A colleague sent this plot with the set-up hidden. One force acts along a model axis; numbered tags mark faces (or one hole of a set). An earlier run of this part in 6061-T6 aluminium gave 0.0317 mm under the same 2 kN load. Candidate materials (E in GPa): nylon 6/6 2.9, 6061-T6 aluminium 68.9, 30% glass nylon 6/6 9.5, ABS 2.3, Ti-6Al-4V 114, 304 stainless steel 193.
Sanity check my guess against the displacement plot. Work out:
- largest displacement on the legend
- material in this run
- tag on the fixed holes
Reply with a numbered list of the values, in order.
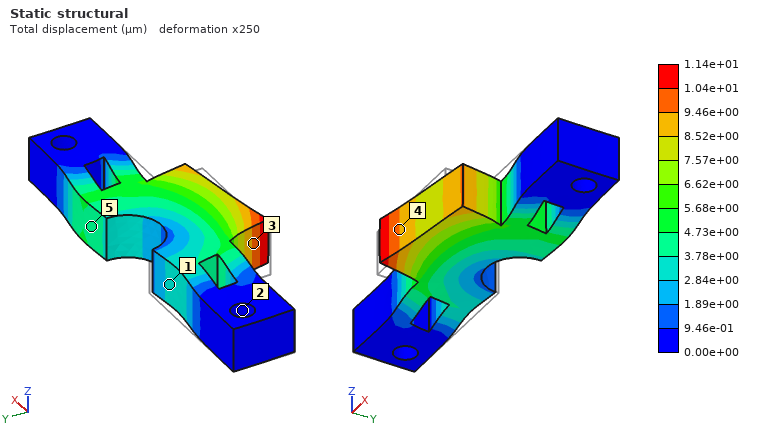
1. 1.14e+01 µm
2. 304 stainless steel
3. 2
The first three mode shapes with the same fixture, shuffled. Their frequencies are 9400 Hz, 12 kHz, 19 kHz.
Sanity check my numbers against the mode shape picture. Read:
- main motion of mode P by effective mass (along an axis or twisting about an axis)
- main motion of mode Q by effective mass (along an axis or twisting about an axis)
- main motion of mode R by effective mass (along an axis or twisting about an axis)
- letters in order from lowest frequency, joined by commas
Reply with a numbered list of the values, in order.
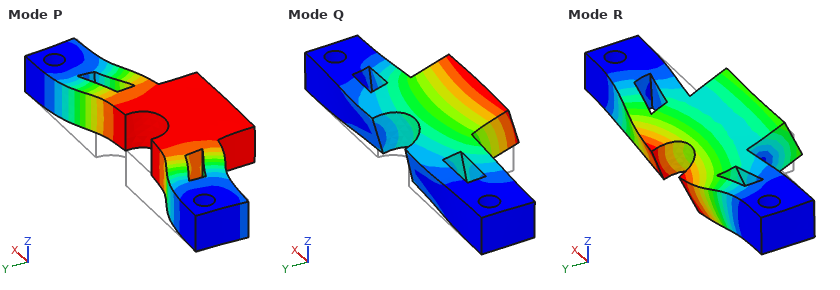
1. along Y
2. along Z
3. along Z
4. Q, P, R
